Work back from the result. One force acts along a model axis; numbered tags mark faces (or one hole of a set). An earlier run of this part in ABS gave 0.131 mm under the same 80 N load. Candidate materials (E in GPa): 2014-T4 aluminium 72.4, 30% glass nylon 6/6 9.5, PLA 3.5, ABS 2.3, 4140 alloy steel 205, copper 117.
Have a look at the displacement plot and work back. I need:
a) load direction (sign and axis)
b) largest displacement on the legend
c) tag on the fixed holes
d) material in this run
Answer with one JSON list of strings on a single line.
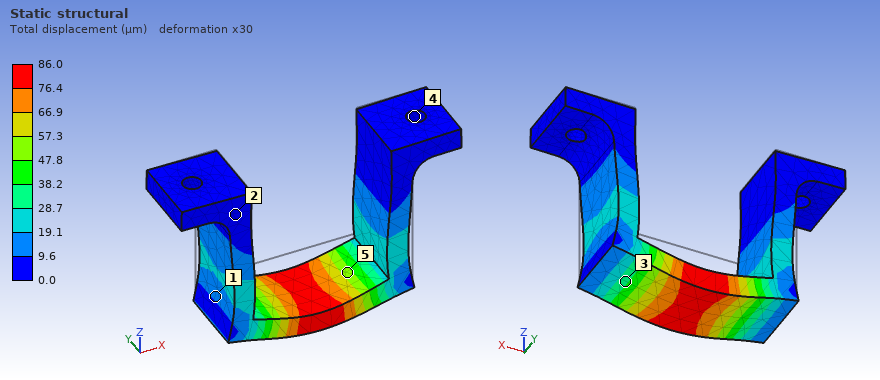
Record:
["-Z", "86.0 µm", "4", "PLA"]
